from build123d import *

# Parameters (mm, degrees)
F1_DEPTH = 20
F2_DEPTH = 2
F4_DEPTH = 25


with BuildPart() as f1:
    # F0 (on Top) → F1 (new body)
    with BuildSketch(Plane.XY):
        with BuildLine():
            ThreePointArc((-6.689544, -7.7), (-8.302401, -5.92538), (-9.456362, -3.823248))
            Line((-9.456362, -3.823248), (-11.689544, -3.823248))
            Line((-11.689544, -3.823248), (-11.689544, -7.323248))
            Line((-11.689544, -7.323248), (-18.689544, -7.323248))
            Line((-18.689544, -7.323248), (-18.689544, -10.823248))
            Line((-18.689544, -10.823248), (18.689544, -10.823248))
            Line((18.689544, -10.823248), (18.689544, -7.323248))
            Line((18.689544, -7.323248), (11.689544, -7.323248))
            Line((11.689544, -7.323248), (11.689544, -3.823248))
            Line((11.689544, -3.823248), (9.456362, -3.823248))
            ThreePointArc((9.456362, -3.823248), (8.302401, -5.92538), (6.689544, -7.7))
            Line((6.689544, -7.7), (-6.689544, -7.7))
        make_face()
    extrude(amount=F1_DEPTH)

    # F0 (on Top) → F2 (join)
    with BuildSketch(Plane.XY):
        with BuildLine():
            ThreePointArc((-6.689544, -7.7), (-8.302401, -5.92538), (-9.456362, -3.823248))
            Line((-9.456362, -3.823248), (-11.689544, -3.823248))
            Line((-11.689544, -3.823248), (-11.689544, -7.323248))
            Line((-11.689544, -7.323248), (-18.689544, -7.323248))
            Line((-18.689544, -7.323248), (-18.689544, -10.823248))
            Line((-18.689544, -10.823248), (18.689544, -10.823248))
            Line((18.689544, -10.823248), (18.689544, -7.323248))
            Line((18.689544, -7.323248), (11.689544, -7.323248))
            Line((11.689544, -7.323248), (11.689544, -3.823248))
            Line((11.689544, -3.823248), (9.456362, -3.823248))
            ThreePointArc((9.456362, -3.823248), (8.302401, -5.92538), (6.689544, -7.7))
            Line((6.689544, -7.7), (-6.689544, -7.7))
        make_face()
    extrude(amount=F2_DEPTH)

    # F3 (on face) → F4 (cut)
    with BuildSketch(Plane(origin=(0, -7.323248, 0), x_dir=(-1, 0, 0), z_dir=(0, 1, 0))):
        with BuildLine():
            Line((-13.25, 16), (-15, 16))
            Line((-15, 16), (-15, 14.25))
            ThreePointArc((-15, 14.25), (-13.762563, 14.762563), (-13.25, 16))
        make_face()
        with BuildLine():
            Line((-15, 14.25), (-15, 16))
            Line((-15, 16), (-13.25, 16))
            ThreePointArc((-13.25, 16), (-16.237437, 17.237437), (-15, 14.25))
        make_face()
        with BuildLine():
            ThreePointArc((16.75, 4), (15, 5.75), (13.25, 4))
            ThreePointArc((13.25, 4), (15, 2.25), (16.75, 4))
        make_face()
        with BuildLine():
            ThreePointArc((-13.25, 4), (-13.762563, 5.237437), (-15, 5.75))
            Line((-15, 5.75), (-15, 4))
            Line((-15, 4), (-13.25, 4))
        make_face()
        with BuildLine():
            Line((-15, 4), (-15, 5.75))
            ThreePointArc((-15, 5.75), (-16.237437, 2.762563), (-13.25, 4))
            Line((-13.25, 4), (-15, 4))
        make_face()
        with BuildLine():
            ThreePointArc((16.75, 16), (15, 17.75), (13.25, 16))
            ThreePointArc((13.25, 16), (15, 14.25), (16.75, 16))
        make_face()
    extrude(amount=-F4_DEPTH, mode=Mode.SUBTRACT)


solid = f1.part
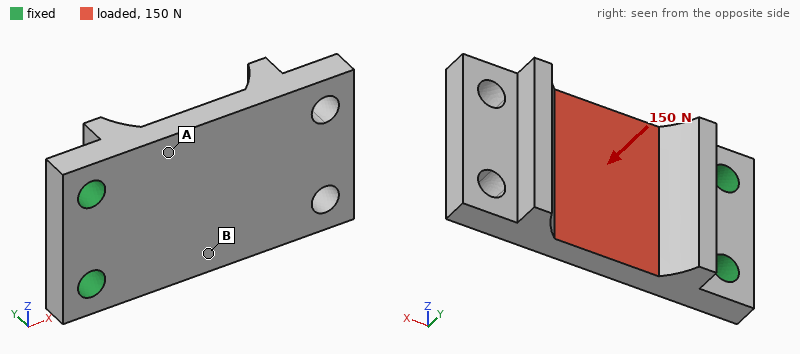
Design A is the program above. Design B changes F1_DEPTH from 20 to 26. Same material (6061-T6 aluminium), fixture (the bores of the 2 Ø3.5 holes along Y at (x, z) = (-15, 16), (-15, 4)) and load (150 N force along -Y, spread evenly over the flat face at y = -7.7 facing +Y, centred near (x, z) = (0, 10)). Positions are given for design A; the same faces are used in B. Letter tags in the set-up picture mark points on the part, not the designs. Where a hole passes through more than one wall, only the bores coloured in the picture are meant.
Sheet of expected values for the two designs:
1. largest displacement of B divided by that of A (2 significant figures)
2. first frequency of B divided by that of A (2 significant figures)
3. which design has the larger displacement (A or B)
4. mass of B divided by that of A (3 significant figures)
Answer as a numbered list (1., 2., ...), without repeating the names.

1. 0.86
2. 0.97
3. A
4. 1.31
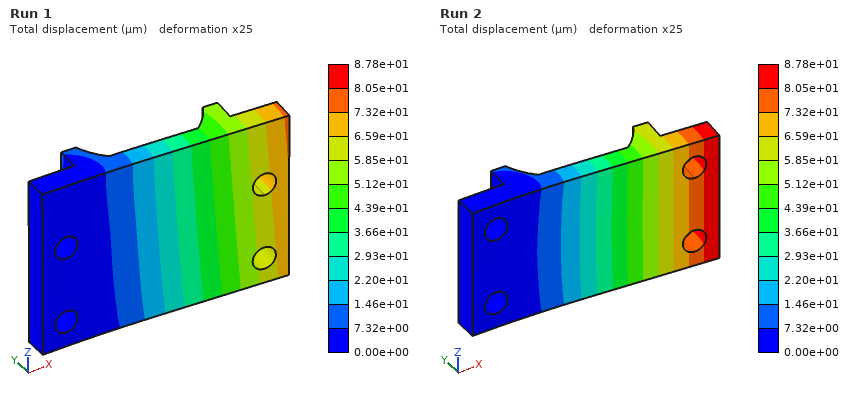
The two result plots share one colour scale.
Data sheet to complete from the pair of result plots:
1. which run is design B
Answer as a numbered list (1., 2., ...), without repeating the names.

1. Run 1
